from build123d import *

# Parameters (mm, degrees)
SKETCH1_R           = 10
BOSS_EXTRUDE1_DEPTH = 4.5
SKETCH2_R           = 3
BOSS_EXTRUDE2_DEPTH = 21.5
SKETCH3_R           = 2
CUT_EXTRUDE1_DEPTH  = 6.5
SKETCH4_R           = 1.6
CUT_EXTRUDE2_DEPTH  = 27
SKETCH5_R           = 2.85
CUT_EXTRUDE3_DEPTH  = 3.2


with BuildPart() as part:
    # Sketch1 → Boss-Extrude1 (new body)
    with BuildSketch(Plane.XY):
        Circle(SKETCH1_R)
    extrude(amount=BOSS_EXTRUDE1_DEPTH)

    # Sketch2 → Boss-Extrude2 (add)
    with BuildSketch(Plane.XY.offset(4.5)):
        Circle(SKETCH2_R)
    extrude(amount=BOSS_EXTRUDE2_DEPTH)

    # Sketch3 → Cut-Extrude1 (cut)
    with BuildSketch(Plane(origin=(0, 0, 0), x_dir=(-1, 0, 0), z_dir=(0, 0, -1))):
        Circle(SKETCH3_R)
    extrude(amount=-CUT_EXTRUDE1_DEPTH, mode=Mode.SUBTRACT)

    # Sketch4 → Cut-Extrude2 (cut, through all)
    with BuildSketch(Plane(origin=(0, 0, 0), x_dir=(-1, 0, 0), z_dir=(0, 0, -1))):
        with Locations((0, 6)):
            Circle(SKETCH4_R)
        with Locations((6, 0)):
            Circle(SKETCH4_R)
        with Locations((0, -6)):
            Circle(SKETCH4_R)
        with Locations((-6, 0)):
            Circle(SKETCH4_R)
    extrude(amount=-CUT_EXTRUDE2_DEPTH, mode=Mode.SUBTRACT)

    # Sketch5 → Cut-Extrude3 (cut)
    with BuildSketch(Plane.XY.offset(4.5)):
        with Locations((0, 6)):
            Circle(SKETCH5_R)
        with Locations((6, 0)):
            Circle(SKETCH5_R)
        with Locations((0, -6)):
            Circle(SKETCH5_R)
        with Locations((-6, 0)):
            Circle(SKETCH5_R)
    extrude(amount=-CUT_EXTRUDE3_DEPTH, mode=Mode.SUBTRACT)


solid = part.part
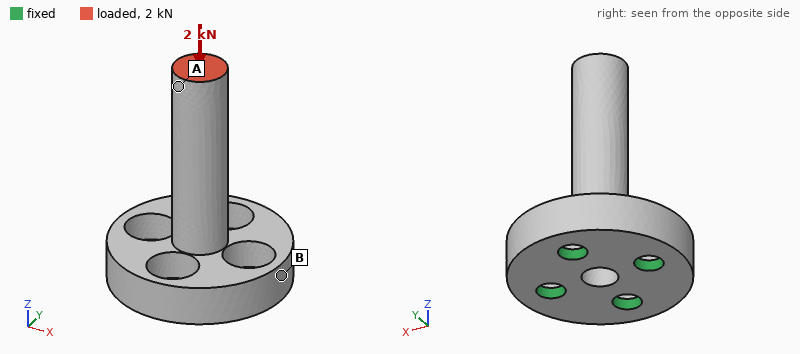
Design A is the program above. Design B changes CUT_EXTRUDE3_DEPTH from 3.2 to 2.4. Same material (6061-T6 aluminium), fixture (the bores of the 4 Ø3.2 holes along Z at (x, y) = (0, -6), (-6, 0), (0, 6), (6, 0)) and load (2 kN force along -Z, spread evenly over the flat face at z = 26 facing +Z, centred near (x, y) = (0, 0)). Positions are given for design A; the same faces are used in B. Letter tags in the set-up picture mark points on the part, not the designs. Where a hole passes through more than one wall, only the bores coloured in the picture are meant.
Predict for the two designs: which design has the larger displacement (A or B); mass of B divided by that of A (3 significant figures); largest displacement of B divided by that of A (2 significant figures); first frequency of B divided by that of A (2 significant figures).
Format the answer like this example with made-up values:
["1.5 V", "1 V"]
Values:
["A", "1.04", "0.92", "1.0"]
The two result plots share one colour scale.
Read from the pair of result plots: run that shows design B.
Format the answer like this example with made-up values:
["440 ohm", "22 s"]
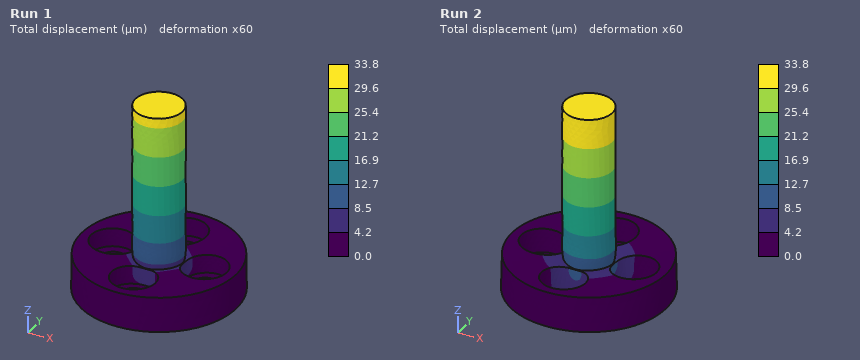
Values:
["Run 1"]
